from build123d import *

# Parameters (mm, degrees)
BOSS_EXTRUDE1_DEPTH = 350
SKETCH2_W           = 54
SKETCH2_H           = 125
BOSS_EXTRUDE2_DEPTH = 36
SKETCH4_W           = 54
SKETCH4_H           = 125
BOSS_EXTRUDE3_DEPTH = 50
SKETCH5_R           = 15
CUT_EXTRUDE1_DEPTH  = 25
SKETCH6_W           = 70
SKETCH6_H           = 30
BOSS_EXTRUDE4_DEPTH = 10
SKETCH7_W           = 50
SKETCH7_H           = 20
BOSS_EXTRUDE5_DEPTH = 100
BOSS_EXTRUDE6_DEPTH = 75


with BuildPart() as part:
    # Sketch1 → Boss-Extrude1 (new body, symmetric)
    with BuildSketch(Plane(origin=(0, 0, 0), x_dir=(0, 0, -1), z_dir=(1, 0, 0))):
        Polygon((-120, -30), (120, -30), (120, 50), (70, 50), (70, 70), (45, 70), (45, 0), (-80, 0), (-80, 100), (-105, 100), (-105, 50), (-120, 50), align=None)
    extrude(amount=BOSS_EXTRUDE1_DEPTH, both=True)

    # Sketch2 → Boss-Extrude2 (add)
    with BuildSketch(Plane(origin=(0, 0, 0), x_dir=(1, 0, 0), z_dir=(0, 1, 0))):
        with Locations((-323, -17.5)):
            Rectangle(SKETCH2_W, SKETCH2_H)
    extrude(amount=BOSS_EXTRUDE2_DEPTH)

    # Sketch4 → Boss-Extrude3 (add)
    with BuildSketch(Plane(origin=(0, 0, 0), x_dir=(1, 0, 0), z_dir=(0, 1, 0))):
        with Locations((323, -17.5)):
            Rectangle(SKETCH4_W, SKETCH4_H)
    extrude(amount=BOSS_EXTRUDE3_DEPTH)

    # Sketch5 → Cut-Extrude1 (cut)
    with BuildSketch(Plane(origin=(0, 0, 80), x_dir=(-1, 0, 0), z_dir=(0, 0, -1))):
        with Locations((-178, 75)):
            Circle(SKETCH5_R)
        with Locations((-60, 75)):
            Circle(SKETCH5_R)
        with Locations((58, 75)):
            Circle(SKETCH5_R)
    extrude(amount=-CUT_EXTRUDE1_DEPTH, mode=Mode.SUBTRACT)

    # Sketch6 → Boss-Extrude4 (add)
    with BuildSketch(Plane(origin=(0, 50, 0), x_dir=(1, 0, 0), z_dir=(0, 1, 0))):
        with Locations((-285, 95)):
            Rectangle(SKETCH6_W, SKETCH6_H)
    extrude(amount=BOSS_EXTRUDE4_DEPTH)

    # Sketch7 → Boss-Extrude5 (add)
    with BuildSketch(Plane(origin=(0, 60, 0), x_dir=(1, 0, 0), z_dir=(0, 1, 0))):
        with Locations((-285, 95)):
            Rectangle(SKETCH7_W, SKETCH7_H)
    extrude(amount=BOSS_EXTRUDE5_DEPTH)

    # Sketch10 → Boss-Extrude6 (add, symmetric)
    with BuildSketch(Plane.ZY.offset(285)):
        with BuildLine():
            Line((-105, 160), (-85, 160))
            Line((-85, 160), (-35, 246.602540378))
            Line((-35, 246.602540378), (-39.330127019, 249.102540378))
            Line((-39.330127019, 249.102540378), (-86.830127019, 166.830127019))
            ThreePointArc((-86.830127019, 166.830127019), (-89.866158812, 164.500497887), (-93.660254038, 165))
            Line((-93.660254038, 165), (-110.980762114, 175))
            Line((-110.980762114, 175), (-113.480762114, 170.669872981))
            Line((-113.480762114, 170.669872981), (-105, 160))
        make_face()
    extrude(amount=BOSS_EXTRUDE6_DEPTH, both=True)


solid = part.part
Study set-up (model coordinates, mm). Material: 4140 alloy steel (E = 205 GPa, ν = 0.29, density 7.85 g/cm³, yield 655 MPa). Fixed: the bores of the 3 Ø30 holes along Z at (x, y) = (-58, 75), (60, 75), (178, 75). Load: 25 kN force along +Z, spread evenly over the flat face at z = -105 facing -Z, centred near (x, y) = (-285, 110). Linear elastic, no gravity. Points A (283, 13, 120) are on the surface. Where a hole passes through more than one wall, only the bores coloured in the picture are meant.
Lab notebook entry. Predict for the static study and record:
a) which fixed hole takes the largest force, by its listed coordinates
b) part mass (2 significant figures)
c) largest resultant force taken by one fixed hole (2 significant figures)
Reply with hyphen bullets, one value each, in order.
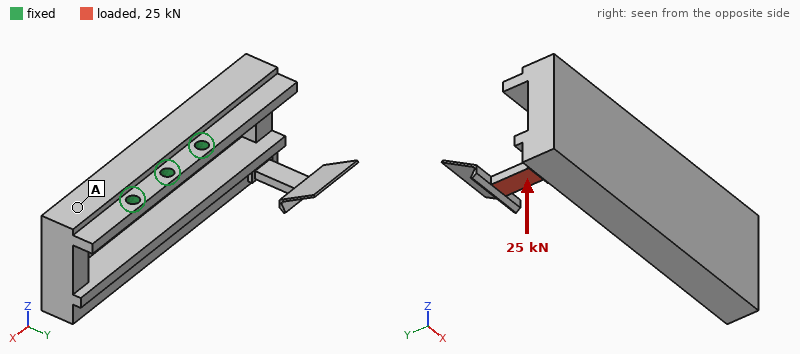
- (-58, 75)
- 87 kg
- 45 kN
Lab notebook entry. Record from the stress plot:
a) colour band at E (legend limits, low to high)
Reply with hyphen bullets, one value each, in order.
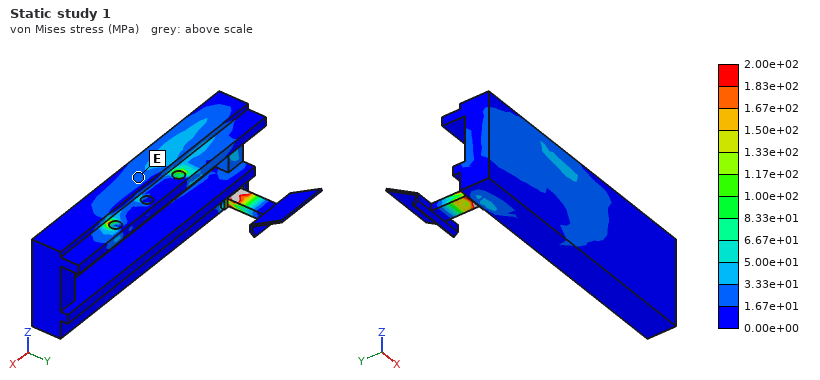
- 1.67e+01 to 3.33e+01 MPa
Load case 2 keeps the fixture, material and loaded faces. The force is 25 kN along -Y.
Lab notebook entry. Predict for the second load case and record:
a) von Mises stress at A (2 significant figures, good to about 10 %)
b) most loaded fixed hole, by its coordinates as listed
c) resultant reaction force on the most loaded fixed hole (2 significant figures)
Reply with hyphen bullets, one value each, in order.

- 20 MPa
- (-58, 75)
- 49 kN
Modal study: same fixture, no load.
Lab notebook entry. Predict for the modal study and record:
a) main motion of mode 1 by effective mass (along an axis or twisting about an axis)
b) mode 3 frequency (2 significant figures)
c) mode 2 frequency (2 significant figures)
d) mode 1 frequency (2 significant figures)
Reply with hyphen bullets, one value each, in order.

- along Y
- 310 Hz
- 270 Hz
- 180 Hz
